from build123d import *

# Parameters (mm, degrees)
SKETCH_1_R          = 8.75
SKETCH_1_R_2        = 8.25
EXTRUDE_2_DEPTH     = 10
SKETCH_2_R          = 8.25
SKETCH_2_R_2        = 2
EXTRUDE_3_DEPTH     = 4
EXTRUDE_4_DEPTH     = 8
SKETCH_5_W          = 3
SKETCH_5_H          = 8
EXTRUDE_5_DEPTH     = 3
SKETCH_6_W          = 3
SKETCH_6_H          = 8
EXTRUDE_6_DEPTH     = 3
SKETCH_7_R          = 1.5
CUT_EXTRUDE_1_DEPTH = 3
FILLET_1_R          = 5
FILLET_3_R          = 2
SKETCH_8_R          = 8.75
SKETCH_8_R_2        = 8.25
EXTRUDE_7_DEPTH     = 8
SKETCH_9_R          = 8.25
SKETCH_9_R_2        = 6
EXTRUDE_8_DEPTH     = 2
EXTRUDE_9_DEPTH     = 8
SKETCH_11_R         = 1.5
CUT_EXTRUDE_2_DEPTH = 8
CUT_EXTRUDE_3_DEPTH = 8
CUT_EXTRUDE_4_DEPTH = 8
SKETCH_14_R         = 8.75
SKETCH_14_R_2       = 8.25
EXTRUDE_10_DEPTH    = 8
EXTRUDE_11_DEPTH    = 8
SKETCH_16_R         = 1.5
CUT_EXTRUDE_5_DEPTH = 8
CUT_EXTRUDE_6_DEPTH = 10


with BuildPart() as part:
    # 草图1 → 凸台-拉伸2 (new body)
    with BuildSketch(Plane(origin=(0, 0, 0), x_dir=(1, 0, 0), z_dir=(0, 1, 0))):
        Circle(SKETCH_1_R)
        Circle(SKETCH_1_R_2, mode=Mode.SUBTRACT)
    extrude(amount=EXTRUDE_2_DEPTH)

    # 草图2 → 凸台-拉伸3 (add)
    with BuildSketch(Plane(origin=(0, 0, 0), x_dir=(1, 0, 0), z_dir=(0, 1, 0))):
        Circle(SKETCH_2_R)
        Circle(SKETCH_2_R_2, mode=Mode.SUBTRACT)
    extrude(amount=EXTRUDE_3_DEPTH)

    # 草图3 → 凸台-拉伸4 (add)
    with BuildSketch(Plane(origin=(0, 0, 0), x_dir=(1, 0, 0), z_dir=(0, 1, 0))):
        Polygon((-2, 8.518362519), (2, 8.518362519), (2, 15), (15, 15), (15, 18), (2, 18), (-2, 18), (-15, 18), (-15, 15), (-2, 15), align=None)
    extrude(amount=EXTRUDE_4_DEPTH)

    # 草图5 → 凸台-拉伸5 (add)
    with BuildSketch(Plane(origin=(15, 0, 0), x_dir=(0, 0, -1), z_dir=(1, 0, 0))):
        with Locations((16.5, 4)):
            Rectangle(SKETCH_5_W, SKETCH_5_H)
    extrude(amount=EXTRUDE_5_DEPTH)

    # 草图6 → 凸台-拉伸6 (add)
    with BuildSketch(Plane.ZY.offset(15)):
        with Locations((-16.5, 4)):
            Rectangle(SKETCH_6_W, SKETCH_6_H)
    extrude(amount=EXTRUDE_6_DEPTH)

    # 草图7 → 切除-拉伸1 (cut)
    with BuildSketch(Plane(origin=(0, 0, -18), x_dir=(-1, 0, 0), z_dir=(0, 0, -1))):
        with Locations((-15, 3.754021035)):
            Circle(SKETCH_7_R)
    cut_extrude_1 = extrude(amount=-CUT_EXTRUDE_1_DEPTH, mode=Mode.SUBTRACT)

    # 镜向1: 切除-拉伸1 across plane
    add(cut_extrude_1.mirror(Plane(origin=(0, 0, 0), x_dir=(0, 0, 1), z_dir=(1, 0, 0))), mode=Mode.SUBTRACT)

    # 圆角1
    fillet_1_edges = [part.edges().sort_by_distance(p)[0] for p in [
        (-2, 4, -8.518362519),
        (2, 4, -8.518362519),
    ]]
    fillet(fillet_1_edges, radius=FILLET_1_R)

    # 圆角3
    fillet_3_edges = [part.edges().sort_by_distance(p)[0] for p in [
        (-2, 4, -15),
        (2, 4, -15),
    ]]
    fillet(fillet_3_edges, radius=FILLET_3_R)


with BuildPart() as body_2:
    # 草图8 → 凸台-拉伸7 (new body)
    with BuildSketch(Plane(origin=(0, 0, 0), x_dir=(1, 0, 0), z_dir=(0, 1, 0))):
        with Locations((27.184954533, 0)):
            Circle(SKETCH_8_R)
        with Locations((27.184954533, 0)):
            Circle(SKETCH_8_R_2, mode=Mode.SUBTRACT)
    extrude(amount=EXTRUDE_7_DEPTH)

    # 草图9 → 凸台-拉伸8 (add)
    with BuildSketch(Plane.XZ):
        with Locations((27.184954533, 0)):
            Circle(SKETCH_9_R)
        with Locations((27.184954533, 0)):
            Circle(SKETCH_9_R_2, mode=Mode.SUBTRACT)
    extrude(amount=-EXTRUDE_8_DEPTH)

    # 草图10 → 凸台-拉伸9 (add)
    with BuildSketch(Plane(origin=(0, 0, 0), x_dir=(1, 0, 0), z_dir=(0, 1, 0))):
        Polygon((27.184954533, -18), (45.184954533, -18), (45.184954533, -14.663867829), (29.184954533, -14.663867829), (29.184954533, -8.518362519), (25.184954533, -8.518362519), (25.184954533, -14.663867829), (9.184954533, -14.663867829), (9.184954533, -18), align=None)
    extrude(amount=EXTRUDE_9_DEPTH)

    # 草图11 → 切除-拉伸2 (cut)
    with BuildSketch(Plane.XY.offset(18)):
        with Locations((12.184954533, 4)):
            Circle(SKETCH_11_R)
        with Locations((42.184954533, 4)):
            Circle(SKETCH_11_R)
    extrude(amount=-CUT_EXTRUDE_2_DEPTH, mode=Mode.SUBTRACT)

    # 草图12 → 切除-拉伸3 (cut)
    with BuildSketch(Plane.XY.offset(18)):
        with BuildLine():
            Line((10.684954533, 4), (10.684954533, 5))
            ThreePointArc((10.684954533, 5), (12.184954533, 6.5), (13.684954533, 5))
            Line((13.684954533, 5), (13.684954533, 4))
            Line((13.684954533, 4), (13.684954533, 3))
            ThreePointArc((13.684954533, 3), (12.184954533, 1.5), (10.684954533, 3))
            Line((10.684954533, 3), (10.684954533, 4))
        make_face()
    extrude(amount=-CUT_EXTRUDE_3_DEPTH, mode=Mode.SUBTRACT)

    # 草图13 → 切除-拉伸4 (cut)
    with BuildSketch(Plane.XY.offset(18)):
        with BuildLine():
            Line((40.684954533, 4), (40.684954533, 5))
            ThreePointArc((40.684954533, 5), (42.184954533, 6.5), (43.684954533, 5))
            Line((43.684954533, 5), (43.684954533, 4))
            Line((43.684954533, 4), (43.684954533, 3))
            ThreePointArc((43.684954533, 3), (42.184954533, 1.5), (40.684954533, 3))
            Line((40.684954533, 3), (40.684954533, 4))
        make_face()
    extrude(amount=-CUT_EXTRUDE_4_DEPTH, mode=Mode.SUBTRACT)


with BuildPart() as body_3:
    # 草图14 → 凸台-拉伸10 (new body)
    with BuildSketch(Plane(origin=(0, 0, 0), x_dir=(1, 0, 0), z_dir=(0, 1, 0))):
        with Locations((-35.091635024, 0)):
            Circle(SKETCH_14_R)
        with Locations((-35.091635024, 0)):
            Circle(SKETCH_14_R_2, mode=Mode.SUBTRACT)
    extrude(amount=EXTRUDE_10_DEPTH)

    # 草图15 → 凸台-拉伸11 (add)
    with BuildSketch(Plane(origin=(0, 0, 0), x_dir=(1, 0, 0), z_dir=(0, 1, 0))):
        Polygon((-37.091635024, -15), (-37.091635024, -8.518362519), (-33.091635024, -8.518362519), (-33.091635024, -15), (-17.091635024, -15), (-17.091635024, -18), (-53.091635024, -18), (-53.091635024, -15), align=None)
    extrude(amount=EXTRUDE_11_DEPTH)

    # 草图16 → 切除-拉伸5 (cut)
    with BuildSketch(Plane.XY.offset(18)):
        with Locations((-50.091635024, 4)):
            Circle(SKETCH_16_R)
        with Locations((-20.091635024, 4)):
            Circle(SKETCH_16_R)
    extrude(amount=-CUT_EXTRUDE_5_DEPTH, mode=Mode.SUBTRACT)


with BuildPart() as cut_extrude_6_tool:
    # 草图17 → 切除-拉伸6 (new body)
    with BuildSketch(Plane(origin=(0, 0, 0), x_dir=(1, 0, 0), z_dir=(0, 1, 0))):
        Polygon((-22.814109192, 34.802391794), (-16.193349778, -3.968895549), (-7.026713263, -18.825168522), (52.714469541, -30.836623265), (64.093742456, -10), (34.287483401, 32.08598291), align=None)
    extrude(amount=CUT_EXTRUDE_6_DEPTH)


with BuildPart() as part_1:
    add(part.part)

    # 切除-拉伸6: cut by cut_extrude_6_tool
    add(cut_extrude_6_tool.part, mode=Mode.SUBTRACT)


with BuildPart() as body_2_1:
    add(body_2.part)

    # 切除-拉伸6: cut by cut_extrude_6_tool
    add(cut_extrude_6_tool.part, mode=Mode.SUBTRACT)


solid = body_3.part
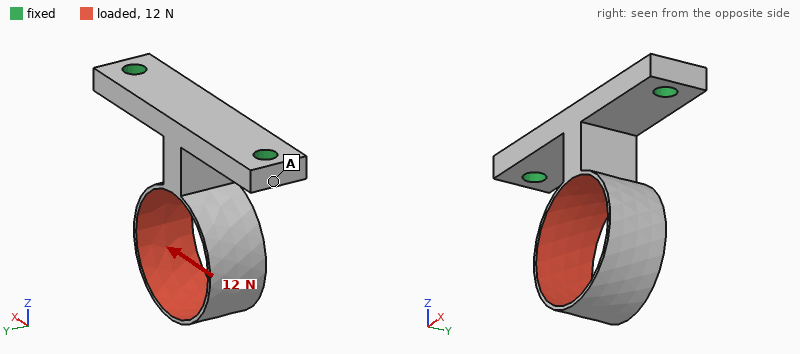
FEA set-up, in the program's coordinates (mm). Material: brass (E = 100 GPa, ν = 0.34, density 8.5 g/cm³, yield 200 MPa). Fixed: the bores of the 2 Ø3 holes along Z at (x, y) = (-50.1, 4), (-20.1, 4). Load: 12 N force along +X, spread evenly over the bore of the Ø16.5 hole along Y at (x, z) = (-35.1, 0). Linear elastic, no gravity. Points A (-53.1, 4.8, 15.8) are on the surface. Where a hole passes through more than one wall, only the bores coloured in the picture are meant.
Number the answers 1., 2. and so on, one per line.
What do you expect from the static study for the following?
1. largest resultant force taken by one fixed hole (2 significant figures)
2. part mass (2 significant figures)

1. 12 N
2. 11 g
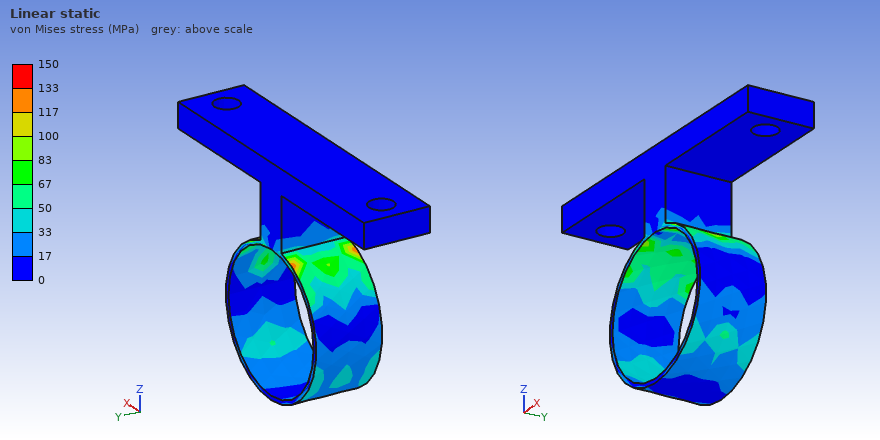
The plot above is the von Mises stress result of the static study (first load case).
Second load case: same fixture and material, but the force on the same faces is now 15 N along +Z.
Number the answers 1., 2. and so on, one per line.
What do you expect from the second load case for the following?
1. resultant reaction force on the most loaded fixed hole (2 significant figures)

1. 7.7 N
